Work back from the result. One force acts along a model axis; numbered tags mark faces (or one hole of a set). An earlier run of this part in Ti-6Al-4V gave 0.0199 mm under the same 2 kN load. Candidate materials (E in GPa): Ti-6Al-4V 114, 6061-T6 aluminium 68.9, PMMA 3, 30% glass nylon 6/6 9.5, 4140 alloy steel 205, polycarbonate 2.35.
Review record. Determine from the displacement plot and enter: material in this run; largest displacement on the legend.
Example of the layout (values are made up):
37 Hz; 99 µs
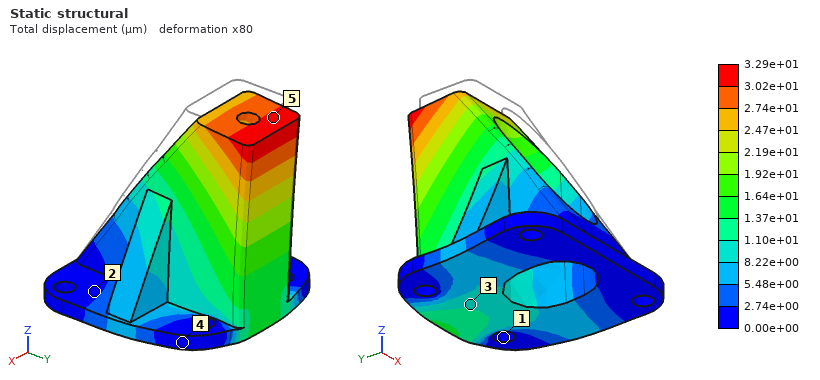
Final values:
6061-T6 aluminium; 3.29e+01 µm
